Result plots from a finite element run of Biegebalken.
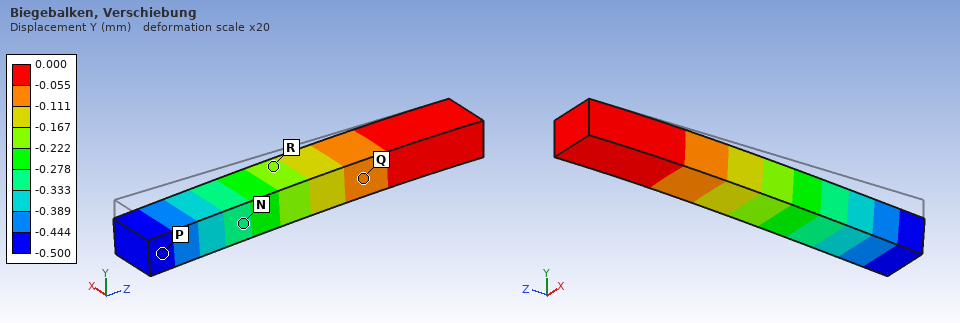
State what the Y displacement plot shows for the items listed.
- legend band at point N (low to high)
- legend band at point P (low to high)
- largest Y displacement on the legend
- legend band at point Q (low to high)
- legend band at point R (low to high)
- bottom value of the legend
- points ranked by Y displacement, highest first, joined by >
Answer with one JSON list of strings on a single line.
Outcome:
["-0.333 to -0.278 mm", "-0.500 to -0.444 mm", "0.000 mm", "-0.111 to -0.055 mm", "-0.222 to -0.167 mm", "-0.500 mm", "Q > R > N > P"]
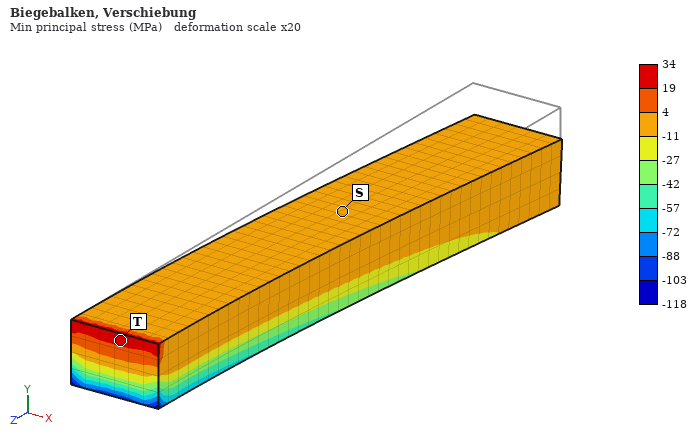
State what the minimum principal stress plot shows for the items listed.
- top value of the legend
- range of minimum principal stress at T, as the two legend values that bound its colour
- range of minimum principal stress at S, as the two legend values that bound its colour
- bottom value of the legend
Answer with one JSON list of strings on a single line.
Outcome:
["34 MPa", "19 to 34 MPa", "-11 to 4 MPa", "-118 MPa"]
